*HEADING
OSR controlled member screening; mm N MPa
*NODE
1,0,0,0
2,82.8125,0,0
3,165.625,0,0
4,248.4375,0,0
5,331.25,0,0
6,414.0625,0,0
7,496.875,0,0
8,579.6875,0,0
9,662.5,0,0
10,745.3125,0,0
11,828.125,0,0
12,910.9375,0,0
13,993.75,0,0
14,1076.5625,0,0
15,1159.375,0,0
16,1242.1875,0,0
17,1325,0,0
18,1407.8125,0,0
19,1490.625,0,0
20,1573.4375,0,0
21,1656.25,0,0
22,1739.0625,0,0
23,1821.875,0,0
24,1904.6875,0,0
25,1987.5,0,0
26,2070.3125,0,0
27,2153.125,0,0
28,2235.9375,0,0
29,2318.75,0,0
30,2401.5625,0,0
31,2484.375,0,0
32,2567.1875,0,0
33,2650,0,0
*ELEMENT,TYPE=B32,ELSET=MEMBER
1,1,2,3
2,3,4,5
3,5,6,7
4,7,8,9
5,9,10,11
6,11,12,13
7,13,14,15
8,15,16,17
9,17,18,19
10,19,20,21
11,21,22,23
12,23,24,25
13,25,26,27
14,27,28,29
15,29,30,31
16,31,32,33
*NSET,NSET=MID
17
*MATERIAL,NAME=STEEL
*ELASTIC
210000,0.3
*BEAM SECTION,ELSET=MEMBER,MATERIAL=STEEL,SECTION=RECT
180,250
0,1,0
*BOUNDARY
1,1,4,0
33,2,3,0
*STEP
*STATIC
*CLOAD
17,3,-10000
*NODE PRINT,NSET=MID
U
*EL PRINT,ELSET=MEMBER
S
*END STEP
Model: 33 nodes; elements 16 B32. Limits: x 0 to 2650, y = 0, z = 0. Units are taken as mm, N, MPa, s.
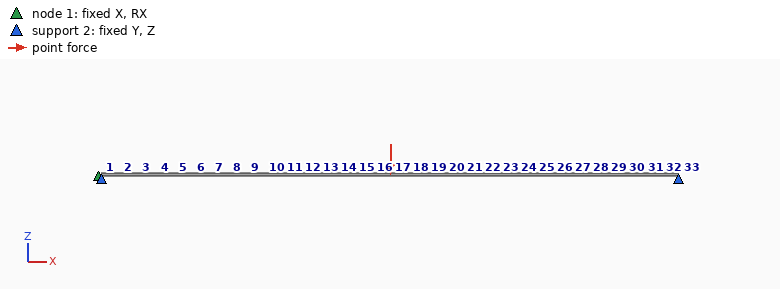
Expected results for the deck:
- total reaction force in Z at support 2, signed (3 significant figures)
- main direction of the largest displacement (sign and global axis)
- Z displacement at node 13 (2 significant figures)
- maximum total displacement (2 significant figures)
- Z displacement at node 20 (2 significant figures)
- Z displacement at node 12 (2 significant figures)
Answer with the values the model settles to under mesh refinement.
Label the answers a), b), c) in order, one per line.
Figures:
a) 10000 N
b) -Z
c) -0.074 mm
d) 0.081 mm
e) -0.077 mm
f) -0.070 mm
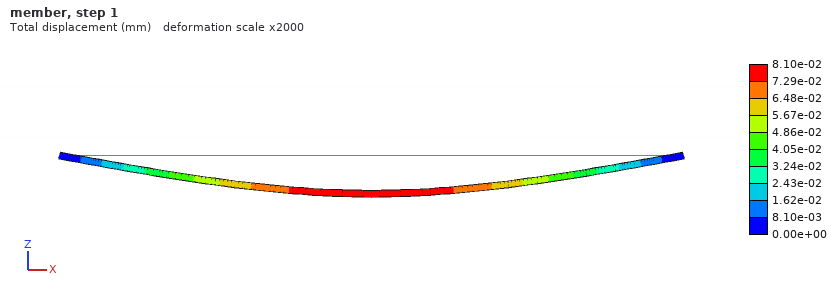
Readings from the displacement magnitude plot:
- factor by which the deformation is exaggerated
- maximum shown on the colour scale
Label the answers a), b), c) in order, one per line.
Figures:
a) 2000
b) 8.10e-02 mm
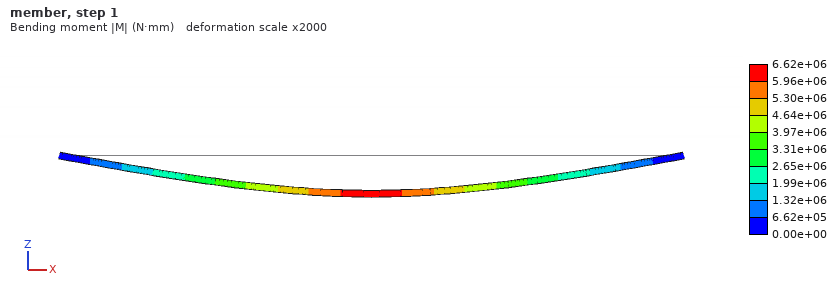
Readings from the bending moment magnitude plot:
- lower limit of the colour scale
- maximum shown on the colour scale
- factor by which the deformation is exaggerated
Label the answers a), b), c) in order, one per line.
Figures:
a) 0.00e+00 N·mm
b) 6.62e+06 N·mm
c) 2000
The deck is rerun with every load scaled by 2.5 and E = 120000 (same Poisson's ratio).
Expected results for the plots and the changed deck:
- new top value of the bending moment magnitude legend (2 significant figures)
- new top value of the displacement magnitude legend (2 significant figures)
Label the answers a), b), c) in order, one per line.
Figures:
a) 1.7e+07 N·mm
b) 0.35 mm
